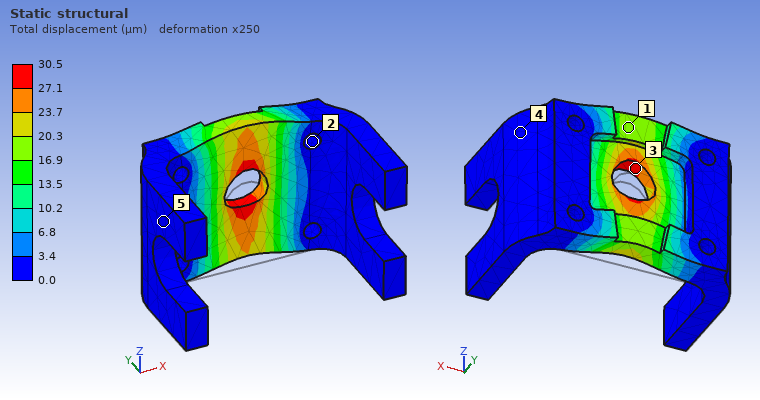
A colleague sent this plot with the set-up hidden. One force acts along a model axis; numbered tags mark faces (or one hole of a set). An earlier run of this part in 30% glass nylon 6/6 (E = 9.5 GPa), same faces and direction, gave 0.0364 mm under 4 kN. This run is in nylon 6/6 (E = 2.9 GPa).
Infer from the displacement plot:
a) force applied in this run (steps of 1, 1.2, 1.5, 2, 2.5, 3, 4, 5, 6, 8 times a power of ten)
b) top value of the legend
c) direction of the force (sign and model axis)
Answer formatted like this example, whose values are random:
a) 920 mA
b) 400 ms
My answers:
a) 1 kN
b) 30.5 µm
c) +Z
